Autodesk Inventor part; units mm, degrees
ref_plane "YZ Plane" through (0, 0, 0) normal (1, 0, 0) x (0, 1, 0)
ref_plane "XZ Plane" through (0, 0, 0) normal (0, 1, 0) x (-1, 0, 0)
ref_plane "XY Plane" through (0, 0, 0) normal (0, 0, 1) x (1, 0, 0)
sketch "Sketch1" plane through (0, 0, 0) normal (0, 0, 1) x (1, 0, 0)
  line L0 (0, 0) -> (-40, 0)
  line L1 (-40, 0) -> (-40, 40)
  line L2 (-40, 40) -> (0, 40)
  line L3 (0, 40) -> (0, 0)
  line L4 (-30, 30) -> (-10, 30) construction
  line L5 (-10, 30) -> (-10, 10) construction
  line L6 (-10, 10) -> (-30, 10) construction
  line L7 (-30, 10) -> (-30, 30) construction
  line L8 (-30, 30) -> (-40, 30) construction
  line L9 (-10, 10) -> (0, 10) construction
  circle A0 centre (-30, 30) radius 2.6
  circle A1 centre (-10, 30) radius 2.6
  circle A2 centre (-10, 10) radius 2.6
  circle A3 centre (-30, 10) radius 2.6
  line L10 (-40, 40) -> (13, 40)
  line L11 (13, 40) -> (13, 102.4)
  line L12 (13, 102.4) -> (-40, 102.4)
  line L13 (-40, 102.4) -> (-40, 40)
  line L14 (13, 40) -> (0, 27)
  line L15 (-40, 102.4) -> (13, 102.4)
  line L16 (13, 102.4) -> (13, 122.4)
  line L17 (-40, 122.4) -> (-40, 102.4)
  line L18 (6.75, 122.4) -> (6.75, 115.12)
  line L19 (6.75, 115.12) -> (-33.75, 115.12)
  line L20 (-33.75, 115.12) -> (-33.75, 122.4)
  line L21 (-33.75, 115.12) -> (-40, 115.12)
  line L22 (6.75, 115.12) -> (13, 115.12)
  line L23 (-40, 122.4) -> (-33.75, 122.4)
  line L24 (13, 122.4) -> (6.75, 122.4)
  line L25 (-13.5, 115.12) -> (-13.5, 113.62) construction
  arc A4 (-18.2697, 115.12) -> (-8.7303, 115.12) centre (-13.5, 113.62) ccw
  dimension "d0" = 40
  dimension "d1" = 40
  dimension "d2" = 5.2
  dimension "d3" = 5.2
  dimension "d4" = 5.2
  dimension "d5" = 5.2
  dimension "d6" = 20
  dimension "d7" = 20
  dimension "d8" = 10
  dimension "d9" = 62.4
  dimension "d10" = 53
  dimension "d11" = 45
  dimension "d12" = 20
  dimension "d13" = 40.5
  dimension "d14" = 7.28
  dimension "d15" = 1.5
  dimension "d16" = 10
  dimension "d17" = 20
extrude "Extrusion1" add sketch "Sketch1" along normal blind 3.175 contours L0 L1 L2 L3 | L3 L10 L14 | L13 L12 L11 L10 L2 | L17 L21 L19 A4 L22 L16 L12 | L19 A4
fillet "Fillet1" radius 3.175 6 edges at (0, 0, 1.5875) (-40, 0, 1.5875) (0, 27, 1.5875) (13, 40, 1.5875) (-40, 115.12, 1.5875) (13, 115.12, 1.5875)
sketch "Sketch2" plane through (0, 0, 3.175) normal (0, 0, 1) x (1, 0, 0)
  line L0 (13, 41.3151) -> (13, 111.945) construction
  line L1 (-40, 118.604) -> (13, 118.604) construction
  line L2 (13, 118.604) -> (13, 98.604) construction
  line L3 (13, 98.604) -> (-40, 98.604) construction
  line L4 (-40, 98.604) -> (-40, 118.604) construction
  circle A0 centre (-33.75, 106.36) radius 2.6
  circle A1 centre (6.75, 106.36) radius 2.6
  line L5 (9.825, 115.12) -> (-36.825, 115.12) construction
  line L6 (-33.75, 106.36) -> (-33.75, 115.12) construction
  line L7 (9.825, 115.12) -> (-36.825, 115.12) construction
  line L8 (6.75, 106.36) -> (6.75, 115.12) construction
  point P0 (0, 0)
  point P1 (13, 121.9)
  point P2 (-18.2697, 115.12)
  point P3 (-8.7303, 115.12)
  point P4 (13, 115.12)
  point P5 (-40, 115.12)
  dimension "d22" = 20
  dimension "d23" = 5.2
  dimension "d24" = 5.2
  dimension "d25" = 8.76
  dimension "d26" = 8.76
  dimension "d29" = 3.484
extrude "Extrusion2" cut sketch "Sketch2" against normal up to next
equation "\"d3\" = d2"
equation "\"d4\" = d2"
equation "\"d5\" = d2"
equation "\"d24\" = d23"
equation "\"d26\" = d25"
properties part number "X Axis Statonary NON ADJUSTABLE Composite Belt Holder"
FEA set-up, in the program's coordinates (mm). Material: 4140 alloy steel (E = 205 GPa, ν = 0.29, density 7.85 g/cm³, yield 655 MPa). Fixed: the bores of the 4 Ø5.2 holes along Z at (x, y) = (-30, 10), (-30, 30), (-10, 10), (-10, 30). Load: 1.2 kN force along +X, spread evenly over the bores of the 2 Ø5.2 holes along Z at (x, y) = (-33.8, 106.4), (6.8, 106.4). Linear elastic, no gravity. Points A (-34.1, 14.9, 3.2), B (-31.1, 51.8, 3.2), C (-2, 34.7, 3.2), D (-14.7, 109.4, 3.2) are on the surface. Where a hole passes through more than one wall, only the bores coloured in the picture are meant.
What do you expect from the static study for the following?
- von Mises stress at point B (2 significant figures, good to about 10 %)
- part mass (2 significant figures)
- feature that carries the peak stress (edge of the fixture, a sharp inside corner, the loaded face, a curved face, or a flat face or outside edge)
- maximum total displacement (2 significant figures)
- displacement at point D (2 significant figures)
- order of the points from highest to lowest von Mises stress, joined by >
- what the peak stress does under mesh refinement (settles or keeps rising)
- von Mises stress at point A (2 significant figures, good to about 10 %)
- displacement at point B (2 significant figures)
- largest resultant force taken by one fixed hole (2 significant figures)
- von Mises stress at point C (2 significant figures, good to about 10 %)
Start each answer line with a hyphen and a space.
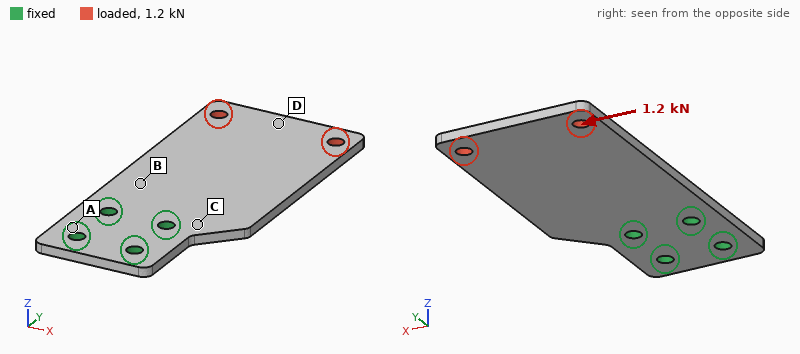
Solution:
- 39 MPa
- 140 g
- edge of the fixture
- 61 µm
- 53 µm
- C > B > A > D
- keeps rising
- 19 MPa
- 12 µm
- 3.1 kN
- 51 MPa
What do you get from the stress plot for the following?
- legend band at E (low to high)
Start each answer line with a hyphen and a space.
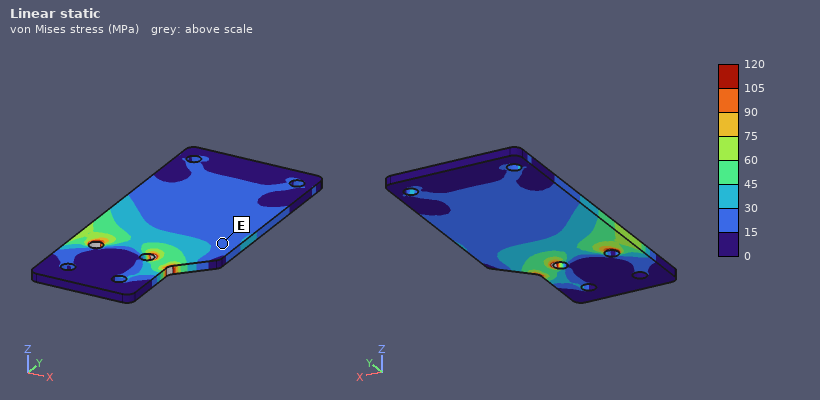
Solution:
- 15 to 30 MPa
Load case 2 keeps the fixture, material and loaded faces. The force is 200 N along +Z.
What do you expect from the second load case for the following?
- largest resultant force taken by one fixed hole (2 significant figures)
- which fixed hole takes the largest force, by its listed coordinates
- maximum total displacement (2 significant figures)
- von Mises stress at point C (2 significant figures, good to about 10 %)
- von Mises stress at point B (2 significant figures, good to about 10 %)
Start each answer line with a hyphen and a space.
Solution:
- 240 N
- (-10, 30)
- 1.2 mm
- 170 MPa
- 130 MPa
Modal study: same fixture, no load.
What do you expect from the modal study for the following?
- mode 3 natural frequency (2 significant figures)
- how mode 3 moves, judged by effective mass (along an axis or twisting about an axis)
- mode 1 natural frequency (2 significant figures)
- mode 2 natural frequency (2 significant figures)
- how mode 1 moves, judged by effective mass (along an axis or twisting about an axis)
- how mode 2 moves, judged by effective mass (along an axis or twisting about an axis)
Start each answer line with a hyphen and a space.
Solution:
- 2200 Hz
- along Z
- 370 Hz
- 1200 Hz
- along Z
- twisting about Y
